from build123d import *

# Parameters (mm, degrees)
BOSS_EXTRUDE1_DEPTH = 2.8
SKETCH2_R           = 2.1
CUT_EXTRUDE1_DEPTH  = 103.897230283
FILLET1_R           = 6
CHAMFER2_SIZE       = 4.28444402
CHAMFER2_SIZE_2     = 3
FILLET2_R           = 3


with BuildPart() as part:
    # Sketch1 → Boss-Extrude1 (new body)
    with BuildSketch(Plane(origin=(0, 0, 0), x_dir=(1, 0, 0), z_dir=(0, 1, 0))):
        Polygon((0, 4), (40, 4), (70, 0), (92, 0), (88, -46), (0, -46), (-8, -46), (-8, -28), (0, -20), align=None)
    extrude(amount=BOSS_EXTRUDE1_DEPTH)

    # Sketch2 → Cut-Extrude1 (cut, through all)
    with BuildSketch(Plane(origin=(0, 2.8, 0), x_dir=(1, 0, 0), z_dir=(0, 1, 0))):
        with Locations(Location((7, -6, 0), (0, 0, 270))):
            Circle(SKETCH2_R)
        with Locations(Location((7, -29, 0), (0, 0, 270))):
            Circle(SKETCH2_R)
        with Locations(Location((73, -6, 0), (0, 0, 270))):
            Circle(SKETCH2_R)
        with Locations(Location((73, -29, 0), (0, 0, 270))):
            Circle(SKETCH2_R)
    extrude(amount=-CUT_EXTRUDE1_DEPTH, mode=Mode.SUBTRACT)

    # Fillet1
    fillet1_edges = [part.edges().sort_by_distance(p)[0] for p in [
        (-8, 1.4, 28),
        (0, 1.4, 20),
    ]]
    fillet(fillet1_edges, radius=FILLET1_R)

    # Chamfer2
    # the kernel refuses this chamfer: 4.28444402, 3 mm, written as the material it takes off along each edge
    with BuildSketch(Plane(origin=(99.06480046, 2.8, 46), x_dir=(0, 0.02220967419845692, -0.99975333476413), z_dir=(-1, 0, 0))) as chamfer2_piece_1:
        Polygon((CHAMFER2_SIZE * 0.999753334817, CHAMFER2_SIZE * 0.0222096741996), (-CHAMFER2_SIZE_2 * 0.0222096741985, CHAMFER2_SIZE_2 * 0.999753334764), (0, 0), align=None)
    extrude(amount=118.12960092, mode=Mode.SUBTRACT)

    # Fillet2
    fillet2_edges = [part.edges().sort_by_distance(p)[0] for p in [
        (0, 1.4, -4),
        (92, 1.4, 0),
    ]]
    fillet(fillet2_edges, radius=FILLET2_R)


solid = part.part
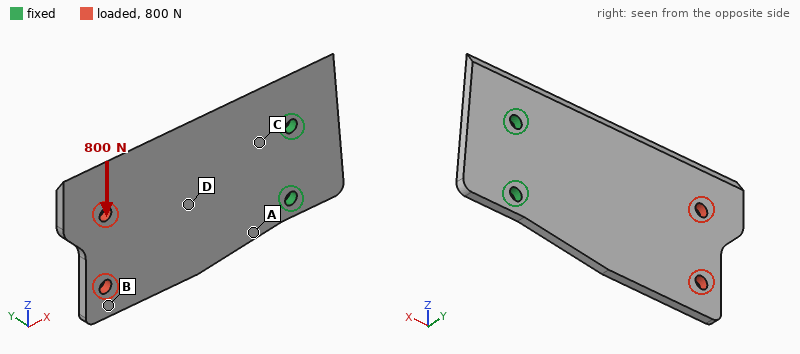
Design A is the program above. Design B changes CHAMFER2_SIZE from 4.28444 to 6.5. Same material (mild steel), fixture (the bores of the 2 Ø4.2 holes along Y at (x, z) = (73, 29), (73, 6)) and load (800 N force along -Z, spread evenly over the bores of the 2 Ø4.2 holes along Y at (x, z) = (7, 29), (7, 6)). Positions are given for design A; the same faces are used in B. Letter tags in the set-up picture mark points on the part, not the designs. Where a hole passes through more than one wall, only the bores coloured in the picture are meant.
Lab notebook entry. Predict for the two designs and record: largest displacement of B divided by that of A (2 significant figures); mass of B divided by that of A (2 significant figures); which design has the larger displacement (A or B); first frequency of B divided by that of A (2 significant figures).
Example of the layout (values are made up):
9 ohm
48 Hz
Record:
1.1
0.97
B
1.0
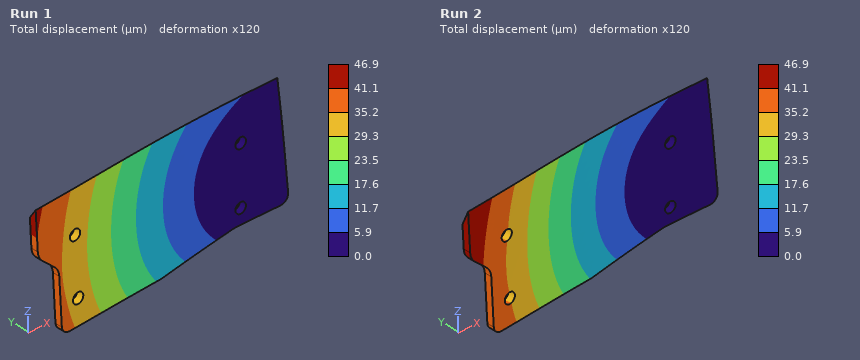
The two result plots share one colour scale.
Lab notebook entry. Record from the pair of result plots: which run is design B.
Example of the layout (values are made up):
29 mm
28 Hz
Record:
Run 2
